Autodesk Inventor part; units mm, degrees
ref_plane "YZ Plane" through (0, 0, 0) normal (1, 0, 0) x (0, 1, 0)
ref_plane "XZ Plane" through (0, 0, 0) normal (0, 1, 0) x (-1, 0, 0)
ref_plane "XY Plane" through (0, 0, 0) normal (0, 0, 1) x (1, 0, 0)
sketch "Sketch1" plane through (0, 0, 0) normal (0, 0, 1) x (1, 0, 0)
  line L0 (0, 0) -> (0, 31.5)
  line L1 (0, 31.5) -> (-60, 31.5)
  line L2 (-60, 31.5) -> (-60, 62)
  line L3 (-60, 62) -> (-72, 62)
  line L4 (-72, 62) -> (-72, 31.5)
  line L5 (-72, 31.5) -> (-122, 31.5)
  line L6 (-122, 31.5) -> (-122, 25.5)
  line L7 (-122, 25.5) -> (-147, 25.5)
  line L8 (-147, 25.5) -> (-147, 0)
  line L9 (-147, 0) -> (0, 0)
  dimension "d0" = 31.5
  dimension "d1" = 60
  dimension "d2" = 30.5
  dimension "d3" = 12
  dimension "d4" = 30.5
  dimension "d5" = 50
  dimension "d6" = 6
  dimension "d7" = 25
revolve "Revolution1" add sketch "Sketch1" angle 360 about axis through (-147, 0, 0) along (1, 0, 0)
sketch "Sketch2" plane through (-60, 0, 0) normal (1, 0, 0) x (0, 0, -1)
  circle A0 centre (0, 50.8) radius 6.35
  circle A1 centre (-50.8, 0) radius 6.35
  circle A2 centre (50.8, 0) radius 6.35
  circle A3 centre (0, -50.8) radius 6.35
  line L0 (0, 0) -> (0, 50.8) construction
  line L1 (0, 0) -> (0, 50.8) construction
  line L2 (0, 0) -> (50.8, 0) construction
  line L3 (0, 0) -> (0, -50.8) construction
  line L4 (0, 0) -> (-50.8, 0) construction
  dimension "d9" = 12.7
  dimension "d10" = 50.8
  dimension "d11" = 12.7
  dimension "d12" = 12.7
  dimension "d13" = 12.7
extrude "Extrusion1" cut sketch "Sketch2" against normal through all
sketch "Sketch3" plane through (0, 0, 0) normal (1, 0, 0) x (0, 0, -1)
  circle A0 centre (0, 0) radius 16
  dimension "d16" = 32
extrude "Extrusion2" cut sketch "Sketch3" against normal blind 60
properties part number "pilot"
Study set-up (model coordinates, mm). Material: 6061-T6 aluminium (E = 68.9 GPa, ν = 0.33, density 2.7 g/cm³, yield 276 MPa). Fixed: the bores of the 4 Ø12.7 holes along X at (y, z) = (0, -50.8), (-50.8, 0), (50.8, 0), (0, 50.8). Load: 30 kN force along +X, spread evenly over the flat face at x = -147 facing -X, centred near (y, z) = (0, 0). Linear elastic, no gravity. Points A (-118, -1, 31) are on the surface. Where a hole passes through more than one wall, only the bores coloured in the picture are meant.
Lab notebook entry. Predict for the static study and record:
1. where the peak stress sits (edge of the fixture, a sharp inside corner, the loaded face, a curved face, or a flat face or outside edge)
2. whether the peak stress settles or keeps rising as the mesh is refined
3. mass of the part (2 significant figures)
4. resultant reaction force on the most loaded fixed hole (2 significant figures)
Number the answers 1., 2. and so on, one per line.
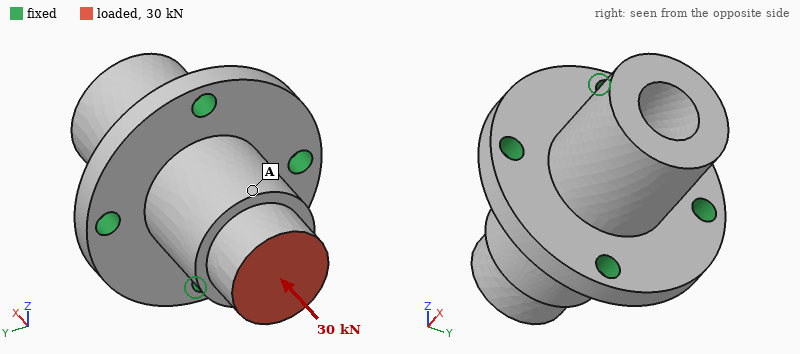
1. edge of the fixture
2. keeps rising
3. 1.3 kg
4. 7.6 kN
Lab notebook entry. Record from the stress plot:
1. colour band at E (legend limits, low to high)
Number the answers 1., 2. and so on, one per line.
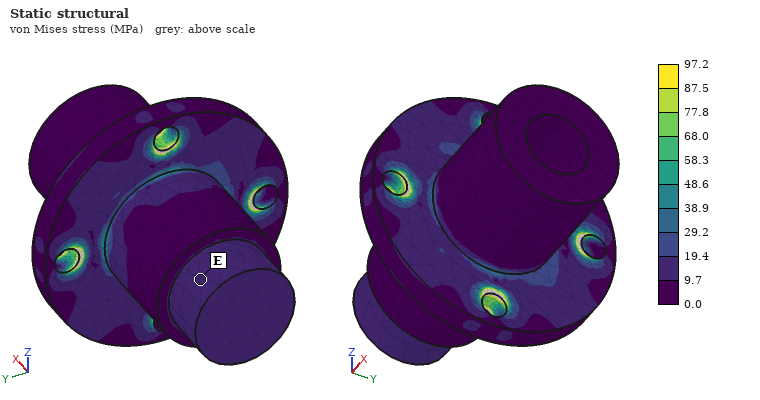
1. 9.7 to 19.4 MPa
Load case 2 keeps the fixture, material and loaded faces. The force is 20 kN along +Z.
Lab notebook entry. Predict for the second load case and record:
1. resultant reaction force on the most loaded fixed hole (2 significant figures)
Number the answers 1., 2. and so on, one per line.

1. 19 kN
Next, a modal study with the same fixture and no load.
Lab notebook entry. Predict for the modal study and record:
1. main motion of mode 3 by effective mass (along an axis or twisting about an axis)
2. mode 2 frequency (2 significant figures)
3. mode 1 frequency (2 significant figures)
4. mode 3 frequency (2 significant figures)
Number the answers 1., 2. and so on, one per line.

1. along X
2. 3100 Hz
3. 3100 Hz
4. 4900 Hz
